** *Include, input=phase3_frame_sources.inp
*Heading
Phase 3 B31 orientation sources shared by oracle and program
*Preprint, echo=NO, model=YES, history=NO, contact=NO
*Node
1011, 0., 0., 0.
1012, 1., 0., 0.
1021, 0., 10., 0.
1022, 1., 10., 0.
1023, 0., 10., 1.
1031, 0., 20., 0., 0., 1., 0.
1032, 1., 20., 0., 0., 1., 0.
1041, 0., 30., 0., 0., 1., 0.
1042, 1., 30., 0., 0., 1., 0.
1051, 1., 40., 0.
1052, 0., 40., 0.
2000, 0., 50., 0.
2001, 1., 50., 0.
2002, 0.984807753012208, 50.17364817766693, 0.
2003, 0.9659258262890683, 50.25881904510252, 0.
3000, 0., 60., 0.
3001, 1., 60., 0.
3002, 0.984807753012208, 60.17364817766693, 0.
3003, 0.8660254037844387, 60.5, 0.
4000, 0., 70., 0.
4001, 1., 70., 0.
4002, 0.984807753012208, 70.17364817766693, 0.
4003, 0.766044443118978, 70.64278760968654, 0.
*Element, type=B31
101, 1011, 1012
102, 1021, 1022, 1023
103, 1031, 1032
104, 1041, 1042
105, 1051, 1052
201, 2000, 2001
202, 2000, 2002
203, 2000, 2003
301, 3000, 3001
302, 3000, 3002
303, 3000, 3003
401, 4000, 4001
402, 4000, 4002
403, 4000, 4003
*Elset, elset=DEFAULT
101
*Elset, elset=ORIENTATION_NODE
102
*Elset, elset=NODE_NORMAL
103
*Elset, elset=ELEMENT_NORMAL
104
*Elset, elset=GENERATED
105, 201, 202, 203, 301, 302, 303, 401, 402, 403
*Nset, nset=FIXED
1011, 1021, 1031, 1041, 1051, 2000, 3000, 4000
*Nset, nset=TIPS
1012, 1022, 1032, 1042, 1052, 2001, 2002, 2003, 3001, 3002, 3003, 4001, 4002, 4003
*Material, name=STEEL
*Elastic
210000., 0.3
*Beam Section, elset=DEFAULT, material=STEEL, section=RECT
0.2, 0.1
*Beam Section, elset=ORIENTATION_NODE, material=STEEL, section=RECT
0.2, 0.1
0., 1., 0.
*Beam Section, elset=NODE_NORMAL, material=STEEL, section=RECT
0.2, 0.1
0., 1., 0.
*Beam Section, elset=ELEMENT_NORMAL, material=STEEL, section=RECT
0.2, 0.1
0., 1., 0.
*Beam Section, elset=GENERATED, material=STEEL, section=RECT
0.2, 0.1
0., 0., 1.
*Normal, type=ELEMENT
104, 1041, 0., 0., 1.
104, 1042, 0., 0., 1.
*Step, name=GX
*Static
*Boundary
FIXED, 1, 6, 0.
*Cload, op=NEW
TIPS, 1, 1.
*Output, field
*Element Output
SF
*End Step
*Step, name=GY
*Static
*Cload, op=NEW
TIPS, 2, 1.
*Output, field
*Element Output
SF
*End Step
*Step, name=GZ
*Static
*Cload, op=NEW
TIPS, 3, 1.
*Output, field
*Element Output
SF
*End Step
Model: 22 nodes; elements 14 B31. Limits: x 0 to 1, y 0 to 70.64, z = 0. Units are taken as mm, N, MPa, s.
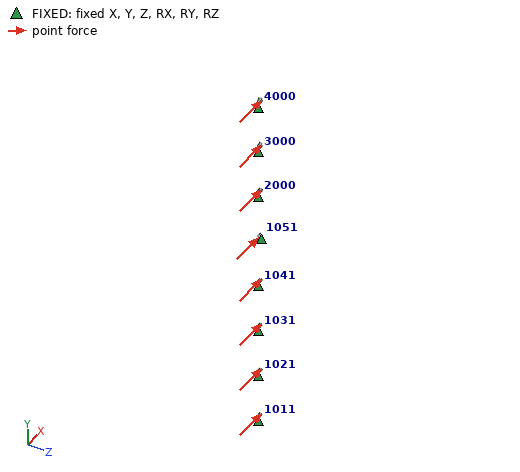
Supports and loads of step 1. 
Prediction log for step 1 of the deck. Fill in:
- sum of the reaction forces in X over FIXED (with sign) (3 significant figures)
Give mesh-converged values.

-14.0 N
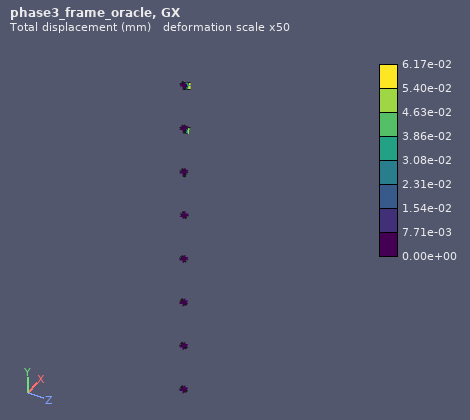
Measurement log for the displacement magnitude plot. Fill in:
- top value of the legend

6.17e-02 mm
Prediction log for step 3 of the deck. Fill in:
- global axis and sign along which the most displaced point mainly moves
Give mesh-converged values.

+Z
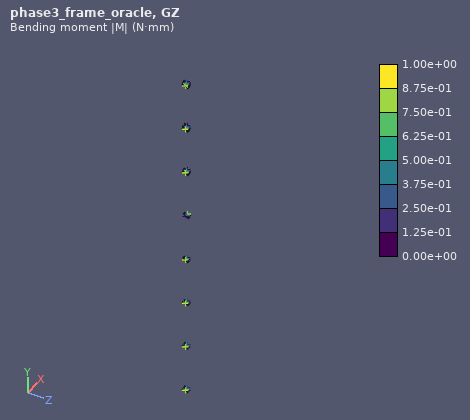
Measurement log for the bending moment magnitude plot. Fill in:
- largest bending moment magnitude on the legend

1.00e+00 N·mm
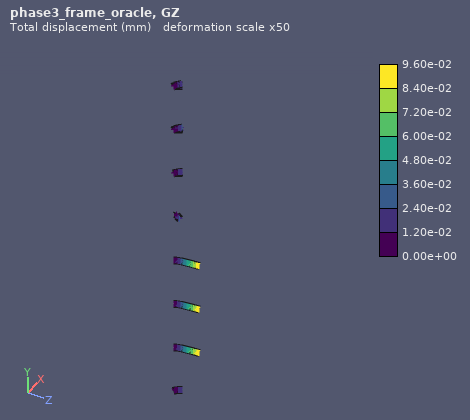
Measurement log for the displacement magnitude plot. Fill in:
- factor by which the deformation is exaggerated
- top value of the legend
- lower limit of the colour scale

50
9.60e-02 mm
0.00e+00 mm
